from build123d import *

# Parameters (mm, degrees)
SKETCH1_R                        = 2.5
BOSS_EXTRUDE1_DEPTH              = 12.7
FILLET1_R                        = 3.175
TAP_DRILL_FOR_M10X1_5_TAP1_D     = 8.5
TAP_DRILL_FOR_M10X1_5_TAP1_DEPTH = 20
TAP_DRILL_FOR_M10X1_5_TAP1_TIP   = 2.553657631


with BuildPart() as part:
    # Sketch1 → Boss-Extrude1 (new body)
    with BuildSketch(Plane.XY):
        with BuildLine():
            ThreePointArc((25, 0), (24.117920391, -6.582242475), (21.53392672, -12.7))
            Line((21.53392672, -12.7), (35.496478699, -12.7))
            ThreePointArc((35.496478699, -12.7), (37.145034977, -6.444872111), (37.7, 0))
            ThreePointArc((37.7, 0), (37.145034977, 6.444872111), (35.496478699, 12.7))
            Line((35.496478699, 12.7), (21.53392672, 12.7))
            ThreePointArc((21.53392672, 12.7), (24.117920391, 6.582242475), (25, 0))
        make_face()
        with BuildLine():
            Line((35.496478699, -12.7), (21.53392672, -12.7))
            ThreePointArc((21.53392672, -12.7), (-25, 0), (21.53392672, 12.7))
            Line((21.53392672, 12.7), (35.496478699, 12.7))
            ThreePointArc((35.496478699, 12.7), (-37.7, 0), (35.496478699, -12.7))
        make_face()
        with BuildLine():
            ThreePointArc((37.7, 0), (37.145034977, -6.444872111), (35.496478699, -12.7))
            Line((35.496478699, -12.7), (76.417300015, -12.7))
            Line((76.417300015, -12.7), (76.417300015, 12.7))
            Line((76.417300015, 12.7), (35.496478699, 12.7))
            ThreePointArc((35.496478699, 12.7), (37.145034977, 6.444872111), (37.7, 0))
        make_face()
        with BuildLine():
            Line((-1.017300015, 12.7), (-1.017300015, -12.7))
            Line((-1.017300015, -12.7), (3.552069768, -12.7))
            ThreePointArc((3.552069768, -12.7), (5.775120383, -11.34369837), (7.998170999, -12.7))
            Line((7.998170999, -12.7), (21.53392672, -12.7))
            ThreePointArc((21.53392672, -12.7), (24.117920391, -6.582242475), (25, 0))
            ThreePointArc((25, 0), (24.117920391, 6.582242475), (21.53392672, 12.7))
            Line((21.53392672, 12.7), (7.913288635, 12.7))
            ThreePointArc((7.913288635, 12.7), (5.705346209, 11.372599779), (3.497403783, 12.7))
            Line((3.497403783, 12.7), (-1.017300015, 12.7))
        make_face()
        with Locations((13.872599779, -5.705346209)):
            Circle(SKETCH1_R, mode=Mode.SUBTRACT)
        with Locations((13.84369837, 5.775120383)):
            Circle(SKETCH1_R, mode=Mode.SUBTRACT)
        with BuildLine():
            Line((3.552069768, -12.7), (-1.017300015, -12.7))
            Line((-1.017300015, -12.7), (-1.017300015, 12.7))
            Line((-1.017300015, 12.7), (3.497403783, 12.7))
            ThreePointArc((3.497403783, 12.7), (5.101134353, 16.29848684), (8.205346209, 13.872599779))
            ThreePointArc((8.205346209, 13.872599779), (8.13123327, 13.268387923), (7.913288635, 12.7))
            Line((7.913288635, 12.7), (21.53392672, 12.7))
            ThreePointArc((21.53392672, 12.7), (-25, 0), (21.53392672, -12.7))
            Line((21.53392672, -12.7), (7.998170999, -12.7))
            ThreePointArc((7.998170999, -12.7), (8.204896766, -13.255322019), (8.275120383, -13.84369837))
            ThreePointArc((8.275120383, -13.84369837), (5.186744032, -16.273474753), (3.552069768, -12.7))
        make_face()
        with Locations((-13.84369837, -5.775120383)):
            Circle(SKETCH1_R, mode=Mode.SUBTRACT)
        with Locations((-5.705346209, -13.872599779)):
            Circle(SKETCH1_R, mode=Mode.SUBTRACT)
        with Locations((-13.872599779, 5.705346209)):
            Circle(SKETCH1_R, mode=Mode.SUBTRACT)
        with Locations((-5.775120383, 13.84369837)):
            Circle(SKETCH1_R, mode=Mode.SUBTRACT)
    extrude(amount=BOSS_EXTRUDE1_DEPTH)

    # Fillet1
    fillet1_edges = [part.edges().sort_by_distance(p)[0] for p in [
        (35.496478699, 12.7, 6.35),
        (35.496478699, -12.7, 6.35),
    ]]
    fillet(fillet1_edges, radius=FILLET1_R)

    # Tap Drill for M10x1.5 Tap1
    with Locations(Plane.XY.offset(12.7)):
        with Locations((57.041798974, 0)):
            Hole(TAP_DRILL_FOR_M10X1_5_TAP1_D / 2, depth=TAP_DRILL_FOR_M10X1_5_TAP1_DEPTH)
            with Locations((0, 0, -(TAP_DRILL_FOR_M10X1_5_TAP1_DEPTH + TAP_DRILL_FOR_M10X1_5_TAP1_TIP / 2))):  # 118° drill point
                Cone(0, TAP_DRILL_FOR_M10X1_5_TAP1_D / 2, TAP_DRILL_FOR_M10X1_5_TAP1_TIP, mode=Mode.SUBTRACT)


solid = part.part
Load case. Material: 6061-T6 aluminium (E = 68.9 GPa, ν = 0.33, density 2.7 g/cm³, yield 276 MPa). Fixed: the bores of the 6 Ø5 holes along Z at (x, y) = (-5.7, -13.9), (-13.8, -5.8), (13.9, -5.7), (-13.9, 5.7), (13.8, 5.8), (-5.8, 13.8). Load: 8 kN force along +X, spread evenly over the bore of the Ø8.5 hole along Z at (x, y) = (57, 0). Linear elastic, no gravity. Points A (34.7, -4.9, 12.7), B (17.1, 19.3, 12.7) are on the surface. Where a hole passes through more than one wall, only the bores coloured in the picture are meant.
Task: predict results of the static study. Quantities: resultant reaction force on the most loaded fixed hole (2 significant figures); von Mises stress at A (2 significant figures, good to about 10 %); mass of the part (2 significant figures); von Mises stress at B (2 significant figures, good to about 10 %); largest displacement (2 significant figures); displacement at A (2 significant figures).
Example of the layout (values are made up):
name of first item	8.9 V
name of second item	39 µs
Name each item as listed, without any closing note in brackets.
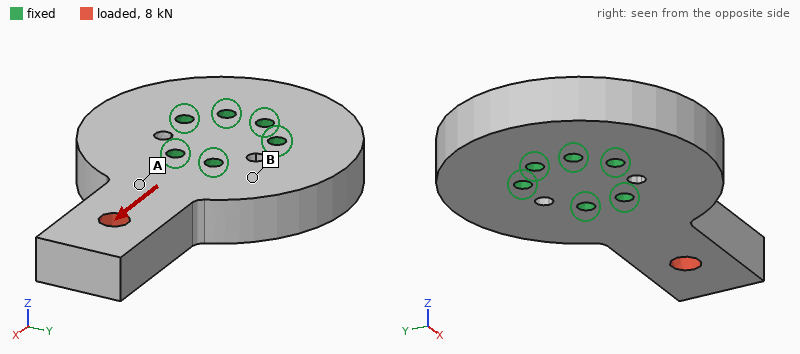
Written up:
resultant reaction force on the most loaded fixed hole	3.3 kN
von Mises stress at A	21 MPa
mass of the part	180 g
von Mises stress at B	6.1 MPa
largest displacement	18 µm
displacement at A	6.2 µm
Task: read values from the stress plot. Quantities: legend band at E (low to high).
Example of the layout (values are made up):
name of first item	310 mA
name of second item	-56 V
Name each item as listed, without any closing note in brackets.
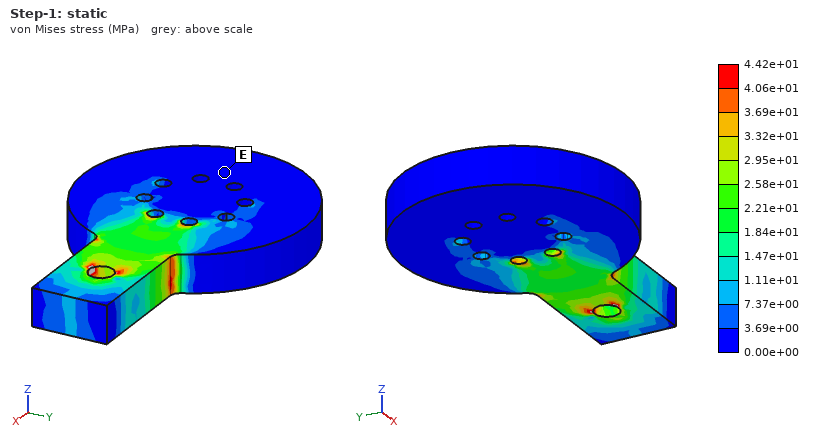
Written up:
legend band at E	0.00e+00 to 3.69e+00 MPa
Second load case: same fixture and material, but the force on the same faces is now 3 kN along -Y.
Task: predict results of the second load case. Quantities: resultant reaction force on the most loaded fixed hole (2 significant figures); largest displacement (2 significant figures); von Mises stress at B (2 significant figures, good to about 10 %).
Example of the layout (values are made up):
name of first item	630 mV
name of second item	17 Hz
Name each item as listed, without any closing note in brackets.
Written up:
resultant reaction force on the most loaded fixed hole	3.2 kN
largest displacement	70 µm
von Mises stress at B	13 MPa
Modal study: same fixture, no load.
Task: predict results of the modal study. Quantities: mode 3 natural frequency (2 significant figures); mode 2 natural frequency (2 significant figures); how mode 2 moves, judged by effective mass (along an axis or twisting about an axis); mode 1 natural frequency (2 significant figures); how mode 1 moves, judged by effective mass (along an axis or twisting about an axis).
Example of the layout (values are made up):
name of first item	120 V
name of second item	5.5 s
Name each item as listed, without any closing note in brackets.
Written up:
mode 3 natural frequency	10 kHz
mode 2 natural frequency	6600 Hz
how mode 2 moves, judged by effective mass	along Y
mode 1 natural frequency	3100 Hz
how mode 1 moves, judged by effective mass	along Z
